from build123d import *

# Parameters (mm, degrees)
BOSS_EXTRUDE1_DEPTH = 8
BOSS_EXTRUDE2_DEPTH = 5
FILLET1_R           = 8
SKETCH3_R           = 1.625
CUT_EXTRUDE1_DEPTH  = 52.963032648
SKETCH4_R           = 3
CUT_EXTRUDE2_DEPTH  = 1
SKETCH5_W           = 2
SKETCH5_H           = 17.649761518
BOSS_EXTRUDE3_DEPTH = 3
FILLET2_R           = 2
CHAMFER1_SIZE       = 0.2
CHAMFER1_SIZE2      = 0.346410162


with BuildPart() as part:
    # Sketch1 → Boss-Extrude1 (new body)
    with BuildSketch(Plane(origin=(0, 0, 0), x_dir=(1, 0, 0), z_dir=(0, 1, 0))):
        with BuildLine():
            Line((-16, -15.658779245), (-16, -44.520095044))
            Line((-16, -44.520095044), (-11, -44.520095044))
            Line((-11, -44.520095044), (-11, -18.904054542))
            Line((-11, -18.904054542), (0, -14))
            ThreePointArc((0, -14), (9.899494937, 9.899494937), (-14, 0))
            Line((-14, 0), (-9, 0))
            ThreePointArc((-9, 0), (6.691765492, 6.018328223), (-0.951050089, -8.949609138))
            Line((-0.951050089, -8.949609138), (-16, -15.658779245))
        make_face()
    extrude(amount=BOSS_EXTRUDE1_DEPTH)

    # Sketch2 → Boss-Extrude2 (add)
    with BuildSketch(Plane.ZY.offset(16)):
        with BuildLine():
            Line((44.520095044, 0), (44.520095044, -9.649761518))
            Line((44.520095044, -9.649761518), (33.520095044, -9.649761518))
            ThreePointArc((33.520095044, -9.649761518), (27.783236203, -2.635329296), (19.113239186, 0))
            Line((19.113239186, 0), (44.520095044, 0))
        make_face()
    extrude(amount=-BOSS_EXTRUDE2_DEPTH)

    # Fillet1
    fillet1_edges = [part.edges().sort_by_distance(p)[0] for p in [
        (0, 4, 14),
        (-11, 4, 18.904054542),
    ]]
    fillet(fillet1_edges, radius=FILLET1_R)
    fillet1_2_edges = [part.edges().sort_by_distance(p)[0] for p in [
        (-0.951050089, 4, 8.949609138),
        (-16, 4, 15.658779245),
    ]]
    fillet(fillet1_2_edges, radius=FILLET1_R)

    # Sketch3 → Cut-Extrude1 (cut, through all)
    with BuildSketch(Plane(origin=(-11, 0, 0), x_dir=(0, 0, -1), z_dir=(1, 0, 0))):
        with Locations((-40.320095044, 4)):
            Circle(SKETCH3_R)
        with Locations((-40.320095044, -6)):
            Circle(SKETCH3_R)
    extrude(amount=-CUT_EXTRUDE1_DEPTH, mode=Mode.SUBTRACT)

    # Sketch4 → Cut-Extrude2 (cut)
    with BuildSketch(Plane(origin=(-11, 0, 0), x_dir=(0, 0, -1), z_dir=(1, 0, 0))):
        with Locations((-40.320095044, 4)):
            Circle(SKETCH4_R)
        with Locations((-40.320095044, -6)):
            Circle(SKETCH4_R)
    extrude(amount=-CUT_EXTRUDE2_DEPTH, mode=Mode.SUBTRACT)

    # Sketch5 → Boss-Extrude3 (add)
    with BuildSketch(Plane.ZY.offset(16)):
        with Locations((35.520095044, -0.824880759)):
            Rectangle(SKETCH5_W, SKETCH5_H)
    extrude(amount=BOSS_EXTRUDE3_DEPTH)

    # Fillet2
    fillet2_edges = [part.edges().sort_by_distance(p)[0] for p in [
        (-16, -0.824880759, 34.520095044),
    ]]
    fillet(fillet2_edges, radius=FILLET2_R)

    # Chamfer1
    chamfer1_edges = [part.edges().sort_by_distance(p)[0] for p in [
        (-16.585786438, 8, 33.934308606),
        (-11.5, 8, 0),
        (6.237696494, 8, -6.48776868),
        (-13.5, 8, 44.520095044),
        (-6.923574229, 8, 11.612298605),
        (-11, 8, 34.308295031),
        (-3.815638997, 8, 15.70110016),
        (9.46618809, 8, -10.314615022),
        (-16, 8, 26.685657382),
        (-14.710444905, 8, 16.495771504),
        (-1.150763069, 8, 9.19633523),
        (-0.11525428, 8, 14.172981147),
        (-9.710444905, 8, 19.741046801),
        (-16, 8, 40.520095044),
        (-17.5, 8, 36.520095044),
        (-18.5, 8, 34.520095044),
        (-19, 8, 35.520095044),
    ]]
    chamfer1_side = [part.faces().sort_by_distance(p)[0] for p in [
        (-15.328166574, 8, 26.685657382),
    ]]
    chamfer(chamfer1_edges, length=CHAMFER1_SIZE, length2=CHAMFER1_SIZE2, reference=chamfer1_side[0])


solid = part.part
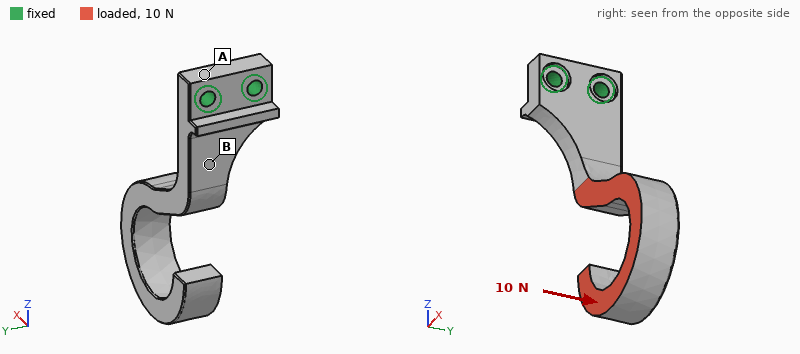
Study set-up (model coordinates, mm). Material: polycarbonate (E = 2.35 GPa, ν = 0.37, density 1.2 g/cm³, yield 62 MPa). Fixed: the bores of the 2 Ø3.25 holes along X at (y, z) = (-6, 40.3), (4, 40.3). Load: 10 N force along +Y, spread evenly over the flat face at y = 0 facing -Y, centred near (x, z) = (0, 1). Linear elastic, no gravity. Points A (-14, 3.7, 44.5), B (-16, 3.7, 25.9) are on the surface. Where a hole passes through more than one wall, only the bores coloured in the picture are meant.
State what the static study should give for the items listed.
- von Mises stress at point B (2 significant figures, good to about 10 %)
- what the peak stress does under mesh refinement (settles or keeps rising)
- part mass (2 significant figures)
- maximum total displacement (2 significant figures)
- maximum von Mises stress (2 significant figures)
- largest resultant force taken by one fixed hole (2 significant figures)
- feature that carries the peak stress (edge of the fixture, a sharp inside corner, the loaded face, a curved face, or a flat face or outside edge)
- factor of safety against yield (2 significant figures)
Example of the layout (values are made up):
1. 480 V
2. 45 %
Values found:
1. 3.7 MPa
2. settles
3. 5.5 g
4. 0.72 mm
5. 7.6 MPa
6. 37 N
7. a curved face
8. 8.1
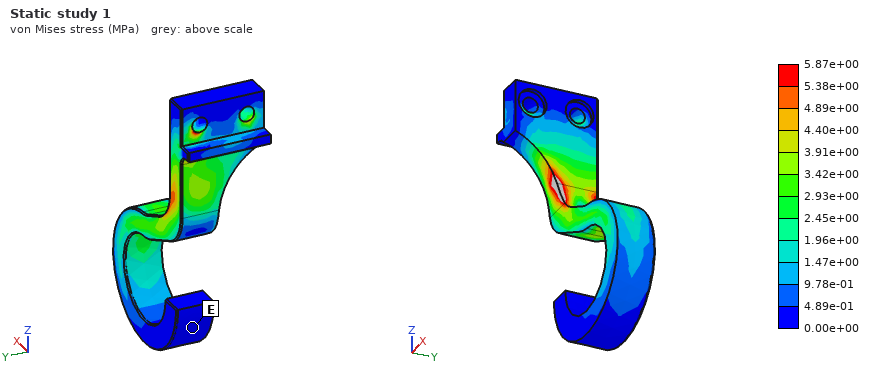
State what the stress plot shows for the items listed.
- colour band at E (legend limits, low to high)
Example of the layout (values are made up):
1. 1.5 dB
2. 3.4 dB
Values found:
1. 0.00e+00 to 4.89e-01 MPa
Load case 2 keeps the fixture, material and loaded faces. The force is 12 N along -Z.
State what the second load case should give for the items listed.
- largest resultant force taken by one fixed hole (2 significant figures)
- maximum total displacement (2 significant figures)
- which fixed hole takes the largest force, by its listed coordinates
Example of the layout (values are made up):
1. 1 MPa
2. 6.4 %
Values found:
1. 7.0 N
2. 0.72 mm
3. (4, 40.3)
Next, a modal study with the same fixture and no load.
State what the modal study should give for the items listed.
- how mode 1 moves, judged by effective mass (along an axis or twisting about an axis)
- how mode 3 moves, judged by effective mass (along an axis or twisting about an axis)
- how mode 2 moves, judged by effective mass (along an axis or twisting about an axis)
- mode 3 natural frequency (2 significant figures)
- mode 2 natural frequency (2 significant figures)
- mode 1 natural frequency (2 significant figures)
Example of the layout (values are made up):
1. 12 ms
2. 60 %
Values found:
1. along X
2. along Z
3. along Y
4. 680 Hz
5. 370 Hz
6. 250 Hz
